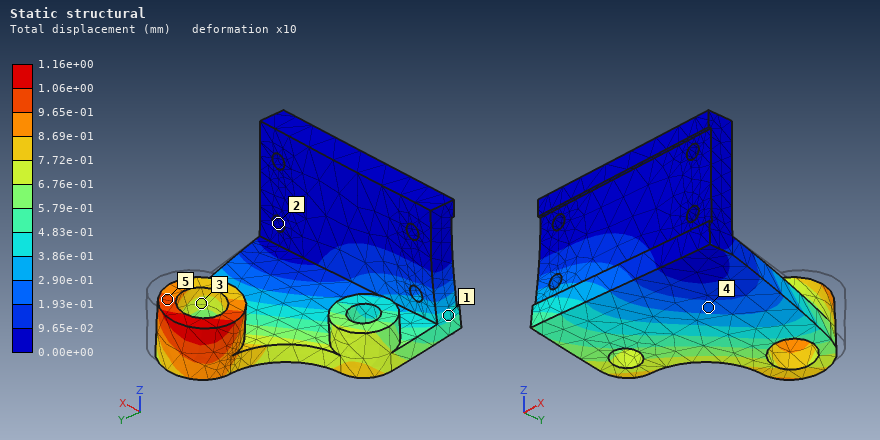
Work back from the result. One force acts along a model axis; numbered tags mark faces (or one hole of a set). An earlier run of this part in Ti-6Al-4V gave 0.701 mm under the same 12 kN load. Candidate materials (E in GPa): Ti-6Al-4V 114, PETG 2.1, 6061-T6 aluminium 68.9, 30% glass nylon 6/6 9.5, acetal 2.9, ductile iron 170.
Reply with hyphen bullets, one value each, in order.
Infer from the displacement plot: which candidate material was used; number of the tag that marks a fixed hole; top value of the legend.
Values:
- 6061-T6 aluminium
- 2
- 1.16e+00 mm
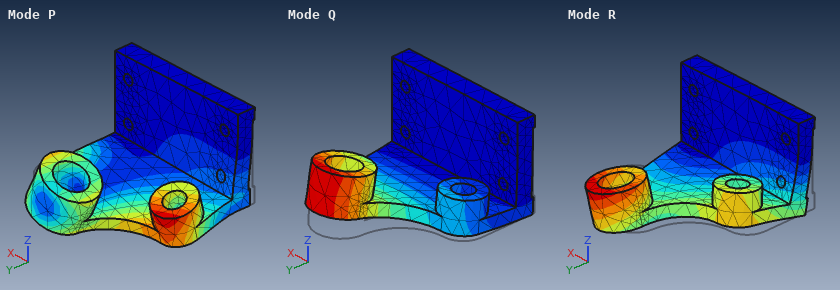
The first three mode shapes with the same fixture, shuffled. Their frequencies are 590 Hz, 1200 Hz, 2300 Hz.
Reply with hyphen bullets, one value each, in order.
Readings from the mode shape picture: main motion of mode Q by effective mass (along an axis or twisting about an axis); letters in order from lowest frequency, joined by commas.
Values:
- along Z
- Q, R, P
